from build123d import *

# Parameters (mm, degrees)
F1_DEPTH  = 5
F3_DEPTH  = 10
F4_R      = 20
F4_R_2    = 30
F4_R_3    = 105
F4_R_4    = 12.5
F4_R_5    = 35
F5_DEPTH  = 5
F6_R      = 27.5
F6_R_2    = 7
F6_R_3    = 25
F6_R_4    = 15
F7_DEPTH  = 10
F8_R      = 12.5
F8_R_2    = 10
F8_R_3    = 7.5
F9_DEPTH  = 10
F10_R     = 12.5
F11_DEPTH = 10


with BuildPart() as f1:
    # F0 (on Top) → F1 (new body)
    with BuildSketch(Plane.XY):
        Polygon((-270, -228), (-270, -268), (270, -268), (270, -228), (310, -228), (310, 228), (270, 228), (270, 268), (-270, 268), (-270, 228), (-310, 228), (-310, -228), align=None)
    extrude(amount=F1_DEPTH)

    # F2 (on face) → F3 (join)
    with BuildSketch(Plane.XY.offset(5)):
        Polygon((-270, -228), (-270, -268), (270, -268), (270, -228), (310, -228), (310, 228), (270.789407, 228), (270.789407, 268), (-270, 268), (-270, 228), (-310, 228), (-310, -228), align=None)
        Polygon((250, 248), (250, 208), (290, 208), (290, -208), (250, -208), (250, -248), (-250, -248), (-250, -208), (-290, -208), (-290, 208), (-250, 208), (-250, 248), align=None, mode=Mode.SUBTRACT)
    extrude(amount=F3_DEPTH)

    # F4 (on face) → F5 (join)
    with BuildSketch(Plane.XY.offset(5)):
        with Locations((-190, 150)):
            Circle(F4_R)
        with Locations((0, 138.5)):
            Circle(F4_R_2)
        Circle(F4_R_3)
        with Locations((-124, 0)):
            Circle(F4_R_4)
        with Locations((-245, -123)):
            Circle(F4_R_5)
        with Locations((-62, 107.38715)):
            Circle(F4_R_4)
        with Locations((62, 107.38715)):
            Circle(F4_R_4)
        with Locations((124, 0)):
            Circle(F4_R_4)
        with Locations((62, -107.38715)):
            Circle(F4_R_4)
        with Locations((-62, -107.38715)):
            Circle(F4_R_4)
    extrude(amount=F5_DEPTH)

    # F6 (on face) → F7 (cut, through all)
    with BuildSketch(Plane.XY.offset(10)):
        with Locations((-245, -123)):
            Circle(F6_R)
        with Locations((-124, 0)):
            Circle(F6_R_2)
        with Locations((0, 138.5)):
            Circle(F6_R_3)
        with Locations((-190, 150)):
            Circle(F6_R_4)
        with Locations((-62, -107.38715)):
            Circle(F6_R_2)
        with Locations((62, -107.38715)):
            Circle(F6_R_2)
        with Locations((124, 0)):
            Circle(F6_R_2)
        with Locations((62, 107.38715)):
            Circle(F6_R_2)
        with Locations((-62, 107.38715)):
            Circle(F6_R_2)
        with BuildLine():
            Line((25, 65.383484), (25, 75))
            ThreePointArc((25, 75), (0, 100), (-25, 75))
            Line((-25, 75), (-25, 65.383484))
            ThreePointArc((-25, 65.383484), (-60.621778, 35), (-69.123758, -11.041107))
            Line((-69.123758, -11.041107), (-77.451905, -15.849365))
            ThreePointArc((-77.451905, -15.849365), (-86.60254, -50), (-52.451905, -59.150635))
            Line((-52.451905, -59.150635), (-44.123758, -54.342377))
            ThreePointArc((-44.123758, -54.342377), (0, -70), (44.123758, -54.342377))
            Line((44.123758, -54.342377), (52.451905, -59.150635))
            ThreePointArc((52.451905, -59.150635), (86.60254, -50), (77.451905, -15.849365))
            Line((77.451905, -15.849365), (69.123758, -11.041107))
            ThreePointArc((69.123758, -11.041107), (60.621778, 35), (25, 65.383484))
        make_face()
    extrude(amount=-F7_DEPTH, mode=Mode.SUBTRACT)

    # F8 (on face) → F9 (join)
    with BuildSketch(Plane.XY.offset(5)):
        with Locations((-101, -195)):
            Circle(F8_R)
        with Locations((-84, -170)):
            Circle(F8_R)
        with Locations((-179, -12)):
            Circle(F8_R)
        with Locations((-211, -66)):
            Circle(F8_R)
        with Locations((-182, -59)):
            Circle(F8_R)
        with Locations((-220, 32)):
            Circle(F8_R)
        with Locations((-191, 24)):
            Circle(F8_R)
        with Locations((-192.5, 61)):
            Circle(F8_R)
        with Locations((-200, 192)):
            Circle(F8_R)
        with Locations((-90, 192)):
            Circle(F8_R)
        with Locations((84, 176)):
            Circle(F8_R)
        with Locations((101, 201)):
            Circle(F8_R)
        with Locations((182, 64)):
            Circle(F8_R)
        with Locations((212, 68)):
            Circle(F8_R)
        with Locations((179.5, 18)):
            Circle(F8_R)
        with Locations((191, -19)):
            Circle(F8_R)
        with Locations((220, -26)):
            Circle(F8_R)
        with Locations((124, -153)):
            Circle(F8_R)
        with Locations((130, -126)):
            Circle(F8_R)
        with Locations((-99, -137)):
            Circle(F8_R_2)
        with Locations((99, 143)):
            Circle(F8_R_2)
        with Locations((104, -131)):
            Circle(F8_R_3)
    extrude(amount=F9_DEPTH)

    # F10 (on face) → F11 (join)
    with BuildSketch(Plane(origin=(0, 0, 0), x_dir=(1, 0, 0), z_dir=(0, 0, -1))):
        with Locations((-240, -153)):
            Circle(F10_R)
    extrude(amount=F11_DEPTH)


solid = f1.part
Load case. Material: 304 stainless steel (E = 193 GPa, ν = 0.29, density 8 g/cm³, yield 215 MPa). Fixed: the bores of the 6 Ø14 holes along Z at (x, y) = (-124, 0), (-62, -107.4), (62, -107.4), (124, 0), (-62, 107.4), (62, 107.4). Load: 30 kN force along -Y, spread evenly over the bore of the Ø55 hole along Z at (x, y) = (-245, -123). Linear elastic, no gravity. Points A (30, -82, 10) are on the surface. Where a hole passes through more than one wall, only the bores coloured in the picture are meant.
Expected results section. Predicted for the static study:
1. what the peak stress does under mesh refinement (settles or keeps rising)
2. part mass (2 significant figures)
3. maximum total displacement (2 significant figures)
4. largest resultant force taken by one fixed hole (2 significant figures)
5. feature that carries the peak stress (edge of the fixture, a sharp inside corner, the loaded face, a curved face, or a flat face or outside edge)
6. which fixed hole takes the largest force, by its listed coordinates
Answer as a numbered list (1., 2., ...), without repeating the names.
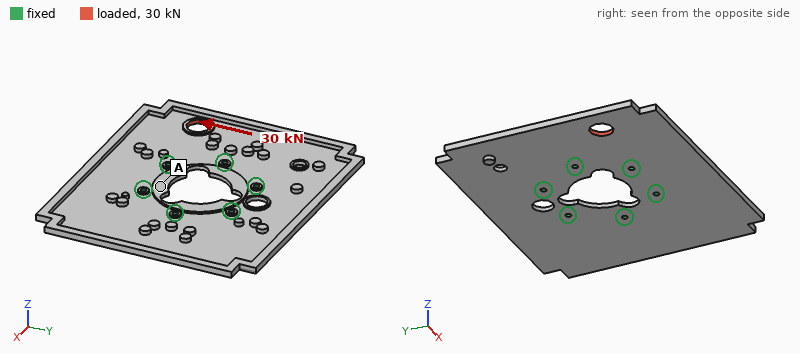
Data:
1. keeps rising
2. 17 kg
3. 0.72 mm
4. 20 kN
5. edge of the fixture
6. (-124, 0)
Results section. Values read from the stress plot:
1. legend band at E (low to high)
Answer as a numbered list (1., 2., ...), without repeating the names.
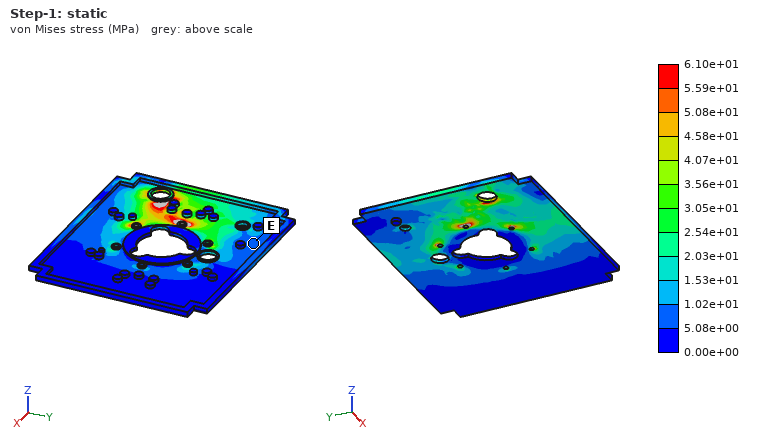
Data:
1. 5.08e+00 to 1.02e+01 MPa
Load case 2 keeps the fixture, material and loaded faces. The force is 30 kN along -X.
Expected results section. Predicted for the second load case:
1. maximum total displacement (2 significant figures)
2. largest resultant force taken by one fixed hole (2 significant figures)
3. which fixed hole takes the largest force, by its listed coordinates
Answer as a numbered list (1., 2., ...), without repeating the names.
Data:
1. 0.86 mm
2. 16 kN
3. (-62, -107.4)
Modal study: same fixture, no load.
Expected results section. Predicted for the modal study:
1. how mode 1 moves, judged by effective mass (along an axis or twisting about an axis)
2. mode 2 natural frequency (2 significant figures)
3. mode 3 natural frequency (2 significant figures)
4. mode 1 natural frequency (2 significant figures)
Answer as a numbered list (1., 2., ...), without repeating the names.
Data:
1. twisting about Y
2. 86 Hz
3. 89 Hz
4. 73 Hz
